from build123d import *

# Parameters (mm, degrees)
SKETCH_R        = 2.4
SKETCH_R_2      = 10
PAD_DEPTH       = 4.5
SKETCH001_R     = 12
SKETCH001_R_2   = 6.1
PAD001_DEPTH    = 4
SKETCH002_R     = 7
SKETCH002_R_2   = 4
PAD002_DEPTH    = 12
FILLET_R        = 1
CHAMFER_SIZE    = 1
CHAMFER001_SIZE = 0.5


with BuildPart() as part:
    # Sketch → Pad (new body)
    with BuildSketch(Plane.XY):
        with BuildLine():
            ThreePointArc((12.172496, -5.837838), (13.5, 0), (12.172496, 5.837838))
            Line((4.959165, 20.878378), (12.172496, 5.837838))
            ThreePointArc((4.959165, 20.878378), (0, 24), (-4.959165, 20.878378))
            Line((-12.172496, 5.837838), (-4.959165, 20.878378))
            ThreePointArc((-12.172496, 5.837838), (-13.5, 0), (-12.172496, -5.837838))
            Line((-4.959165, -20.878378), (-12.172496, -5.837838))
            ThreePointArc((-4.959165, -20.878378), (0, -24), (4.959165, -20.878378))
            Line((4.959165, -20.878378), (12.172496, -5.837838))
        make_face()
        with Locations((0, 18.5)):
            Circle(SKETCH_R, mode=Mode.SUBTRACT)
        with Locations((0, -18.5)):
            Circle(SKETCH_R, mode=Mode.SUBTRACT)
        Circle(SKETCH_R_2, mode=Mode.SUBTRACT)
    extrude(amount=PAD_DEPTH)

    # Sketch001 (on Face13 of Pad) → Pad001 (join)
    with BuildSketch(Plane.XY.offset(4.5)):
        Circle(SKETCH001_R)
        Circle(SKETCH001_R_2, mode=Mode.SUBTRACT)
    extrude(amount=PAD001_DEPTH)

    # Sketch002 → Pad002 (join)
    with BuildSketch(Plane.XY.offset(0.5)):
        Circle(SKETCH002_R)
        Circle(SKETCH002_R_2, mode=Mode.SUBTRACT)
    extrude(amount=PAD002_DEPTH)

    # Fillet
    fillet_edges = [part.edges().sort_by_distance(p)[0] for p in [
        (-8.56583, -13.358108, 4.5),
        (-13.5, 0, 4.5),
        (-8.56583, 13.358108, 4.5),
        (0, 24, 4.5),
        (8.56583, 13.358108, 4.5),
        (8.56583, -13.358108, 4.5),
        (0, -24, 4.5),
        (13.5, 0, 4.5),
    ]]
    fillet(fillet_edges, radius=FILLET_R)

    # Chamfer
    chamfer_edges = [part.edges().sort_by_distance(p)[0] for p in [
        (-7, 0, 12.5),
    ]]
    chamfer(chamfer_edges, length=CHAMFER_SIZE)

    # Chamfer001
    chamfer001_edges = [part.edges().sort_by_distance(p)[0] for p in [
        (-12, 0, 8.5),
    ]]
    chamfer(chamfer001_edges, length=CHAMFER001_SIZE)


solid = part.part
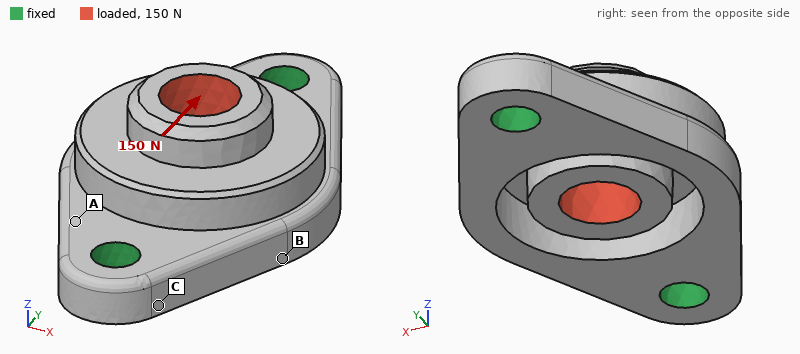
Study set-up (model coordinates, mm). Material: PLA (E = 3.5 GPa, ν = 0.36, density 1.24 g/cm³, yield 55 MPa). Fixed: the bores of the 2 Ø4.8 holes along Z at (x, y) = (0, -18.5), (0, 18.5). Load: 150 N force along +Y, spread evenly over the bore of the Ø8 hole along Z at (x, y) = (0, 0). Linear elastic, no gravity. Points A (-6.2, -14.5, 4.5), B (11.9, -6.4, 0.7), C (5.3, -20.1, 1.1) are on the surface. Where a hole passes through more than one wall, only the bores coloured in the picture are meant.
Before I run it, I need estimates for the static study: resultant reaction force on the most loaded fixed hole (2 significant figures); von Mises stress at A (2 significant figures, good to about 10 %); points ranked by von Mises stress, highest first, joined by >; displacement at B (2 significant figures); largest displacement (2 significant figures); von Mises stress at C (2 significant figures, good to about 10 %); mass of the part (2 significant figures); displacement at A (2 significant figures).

78 N
1.4 MPa
A > C > B
4.7 µm
12 µm
0.83 MPa
5.8 g
3.3 µm
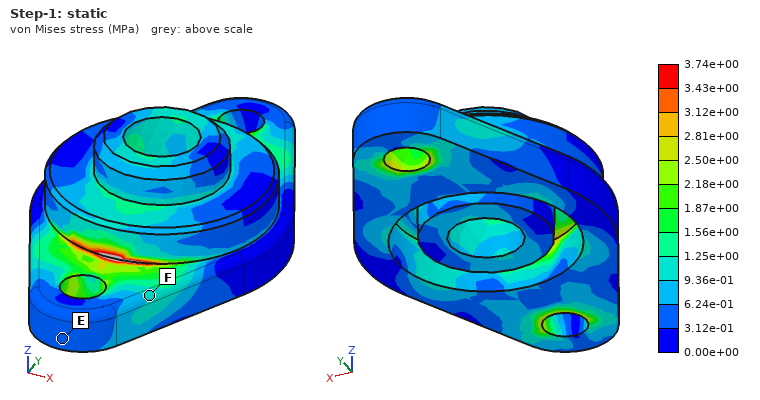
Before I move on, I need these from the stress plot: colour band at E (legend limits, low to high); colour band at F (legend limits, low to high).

3.12e-01 to 6.24e-01 MPa
9.36e-01 to 1.25e+00 MPa
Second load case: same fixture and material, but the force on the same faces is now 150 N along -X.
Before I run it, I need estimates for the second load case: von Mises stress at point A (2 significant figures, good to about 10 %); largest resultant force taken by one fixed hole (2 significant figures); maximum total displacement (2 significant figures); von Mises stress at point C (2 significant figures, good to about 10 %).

4.3 MPa
75 N
66 µm
2.1 MPa
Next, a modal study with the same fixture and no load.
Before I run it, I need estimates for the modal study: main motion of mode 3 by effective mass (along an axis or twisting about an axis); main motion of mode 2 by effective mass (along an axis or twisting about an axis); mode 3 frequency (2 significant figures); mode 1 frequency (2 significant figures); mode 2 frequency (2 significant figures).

along X
along Z
9000 Hz
3600 Hz
5400 Hz
